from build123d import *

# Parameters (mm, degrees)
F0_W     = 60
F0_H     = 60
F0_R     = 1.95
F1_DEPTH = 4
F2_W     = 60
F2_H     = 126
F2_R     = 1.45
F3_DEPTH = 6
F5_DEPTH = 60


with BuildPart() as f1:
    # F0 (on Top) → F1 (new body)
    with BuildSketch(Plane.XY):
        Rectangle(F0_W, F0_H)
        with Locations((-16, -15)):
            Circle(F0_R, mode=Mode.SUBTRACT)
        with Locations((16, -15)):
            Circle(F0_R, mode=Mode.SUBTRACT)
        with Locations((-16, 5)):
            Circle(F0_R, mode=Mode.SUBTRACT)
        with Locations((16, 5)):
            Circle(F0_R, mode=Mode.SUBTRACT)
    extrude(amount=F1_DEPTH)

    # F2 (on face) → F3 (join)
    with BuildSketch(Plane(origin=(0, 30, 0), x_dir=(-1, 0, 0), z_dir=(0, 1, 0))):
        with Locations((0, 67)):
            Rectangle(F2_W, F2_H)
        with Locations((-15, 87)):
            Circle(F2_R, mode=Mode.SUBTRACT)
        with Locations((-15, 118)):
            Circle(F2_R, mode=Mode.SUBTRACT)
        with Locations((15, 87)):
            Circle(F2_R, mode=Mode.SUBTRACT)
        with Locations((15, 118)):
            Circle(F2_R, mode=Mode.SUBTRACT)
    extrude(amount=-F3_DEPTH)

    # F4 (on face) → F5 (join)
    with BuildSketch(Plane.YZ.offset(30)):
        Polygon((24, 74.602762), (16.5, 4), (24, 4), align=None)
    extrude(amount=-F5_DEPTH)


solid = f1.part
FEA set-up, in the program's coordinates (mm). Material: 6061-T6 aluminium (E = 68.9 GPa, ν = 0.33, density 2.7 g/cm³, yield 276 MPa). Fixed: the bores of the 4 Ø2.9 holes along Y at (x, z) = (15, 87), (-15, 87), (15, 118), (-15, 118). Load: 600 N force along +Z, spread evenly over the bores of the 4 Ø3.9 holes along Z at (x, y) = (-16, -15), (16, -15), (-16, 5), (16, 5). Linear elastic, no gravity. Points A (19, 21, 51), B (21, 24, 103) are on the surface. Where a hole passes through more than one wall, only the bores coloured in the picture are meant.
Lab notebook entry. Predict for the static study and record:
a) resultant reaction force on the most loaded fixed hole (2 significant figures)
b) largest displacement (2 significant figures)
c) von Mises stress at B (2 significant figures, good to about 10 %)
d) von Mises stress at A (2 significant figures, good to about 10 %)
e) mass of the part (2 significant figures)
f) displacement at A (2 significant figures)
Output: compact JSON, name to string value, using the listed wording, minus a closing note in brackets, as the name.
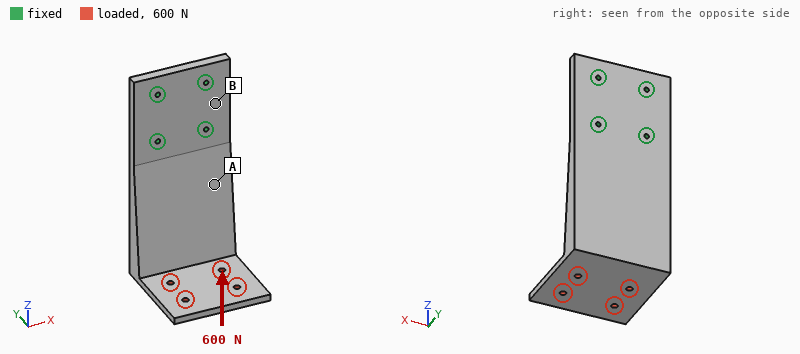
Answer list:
{"resultant reaction force on the most loaded fixed hole": "280 N", "largest displacement": "1.0 mm", "von Mises stress at B": "8.2 MPa", "von Mises stress at A": "26 MPa", "mass of the part": "200 g", "displacement at A": "0.17 mm"}
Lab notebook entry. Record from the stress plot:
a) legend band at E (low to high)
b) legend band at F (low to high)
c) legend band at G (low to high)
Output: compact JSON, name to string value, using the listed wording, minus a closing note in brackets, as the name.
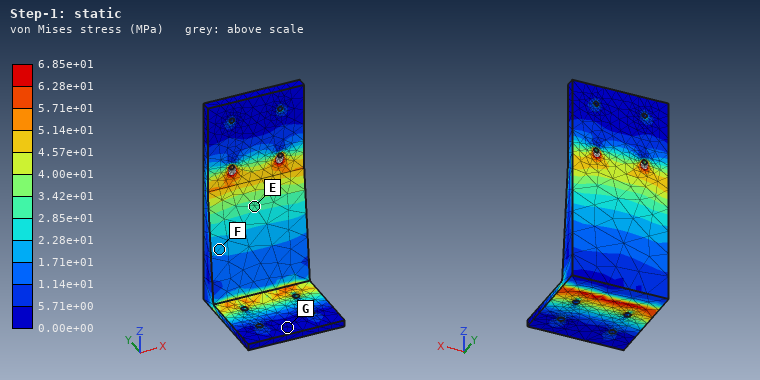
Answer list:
{"legend band at E": "2.85e+01 to 3.42e+01 MPa", "legend band at F": "1.71e+01 to 2.28e+01 MPa", "legend band at G": "0.00e+00 to 5.71e+00 MPa"}
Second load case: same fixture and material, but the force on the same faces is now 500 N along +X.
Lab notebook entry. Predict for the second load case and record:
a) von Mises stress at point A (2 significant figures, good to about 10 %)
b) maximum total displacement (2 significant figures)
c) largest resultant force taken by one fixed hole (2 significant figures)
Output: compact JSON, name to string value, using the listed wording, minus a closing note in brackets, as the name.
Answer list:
{"von Mises stress at point A": "20 MPa", "maximum total displacement": "0.24 mm", "largest resultant force taken by one fixed hole": "1.0 kN"}
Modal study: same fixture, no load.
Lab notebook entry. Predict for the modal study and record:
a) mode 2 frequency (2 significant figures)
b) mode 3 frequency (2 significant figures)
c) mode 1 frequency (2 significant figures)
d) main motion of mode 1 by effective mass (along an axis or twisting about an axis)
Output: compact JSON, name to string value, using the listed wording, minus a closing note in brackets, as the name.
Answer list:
{"mode 2 frequency": "1200 Hz", "mode 3 frequency": "1400 Hz", "mode 1 frequency": "370 Hz", "main motion of mode 1 by effective mass": "along Y"}
